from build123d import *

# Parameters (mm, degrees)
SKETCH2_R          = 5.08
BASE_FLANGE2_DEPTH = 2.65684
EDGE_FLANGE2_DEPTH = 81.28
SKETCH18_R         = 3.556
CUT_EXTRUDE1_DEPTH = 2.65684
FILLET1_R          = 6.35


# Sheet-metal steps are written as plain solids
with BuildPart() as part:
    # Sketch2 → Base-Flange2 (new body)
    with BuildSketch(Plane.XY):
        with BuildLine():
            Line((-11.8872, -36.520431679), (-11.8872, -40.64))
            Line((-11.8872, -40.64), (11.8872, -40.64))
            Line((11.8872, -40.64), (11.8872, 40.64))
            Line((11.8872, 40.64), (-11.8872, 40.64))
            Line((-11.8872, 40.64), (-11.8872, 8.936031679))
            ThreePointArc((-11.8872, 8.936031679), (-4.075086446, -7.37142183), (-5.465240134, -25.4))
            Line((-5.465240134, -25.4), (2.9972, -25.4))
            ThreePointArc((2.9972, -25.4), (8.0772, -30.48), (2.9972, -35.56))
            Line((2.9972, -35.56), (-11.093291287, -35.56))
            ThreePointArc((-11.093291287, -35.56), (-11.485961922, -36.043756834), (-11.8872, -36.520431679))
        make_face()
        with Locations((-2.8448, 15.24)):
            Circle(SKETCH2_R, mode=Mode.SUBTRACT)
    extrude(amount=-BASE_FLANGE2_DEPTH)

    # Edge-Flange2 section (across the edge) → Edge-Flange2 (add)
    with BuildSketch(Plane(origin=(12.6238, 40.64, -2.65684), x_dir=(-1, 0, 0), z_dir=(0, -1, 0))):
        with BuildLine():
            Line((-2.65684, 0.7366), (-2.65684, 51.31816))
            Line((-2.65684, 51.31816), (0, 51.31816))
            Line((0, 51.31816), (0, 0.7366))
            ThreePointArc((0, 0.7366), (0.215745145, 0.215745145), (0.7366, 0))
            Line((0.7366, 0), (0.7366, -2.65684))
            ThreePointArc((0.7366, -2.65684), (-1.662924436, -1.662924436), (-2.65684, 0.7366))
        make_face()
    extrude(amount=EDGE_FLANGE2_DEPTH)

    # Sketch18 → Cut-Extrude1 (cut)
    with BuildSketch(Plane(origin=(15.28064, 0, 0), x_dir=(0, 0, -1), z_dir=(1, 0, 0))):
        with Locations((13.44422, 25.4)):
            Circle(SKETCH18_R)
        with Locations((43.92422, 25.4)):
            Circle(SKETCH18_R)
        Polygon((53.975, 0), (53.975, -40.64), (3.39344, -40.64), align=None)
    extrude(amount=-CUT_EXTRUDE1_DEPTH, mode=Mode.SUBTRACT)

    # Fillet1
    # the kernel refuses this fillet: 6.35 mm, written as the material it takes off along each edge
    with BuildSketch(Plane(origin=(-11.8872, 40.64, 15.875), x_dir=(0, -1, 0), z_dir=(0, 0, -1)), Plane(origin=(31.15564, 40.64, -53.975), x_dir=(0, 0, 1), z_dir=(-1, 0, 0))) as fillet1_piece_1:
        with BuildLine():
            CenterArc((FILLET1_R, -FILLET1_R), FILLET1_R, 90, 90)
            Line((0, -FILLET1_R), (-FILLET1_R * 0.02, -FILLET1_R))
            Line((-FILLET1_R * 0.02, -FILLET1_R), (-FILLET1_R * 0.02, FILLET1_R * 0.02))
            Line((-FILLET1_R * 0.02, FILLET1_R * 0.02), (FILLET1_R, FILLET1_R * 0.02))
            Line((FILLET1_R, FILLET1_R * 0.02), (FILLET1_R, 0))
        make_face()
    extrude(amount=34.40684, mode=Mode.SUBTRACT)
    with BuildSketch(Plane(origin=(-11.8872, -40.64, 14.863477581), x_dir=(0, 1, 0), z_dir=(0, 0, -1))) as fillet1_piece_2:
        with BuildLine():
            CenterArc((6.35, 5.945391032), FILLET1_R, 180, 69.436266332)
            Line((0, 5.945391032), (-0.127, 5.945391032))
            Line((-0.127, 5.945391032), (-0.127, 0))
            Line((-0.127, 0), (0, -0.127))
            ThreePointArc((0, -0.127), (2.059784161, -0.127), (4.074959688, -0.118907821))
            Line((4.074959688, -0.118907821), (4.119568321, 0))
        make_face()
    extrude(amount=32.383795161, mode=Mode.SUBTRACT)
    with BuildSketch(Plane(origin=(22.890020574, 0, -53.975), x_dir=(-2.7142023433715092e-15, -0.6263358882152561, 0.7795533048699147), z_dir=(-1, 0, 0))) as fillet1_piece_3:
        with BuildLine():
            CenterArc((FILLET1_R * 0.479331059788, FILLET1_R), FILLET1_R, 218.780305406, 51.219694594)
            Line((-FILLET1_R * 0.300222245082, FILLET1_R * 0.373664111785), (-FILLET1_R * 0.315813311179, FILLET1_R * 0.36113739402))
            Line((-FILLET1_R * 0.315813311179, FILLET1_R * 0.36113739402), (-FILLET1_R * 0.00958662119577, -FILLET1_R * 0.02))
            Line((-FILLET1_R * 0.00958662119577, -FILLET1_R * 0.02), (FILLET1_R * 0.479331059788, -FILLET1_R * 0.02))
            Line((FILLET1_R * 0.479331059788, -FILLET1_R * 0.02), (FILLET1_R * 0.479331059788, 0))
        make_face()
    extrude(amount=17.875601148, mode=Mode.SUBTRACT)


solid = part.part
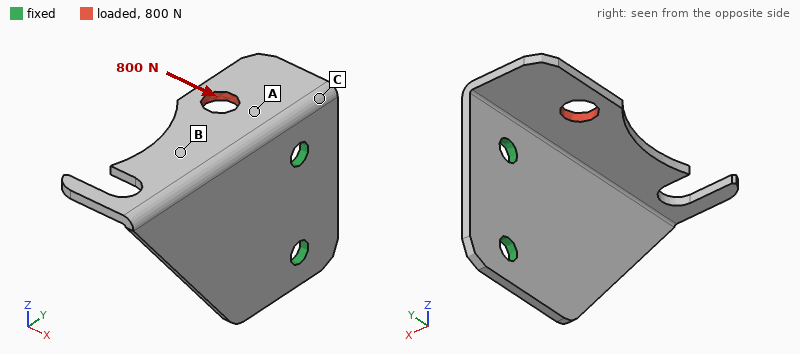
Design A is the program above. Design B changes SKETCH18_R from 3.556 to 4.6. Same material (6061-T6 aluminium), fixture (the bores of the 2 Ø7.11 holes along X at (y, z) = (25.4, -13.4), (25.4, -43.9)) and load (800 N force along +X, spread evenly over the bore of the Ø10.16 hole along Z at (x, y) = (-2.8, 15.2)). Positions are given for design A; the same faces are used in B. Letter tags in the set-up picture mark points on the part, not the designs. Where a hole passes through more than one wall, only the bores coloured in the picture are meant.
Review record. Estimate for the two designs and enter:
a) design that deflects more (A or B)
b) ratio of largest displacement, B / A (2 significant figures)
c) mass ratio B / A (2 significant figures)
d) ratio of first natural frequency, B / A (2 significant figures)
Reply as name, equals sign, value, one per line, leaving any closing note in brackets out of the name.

design that deflects more = A
ratio of largest displacement, B / A = 0.80
mass ratio B / A = 0.99
ratio of first natural frequency, B / A = 1.1
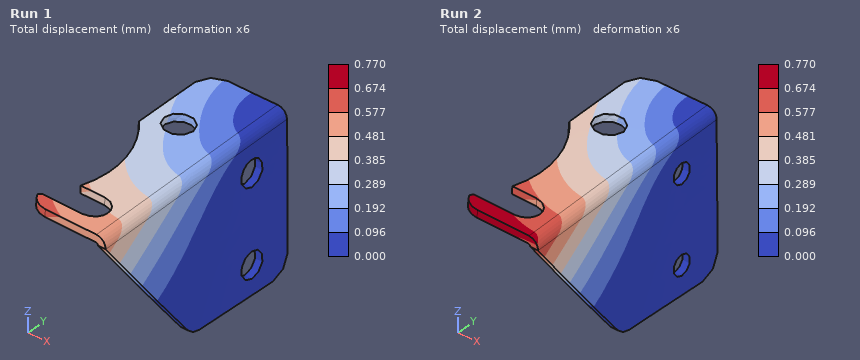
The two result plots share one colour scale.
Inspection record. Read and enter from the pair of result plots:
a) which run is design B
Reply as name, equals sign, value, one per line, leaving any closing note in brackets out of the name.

which run is design B = Run 1
